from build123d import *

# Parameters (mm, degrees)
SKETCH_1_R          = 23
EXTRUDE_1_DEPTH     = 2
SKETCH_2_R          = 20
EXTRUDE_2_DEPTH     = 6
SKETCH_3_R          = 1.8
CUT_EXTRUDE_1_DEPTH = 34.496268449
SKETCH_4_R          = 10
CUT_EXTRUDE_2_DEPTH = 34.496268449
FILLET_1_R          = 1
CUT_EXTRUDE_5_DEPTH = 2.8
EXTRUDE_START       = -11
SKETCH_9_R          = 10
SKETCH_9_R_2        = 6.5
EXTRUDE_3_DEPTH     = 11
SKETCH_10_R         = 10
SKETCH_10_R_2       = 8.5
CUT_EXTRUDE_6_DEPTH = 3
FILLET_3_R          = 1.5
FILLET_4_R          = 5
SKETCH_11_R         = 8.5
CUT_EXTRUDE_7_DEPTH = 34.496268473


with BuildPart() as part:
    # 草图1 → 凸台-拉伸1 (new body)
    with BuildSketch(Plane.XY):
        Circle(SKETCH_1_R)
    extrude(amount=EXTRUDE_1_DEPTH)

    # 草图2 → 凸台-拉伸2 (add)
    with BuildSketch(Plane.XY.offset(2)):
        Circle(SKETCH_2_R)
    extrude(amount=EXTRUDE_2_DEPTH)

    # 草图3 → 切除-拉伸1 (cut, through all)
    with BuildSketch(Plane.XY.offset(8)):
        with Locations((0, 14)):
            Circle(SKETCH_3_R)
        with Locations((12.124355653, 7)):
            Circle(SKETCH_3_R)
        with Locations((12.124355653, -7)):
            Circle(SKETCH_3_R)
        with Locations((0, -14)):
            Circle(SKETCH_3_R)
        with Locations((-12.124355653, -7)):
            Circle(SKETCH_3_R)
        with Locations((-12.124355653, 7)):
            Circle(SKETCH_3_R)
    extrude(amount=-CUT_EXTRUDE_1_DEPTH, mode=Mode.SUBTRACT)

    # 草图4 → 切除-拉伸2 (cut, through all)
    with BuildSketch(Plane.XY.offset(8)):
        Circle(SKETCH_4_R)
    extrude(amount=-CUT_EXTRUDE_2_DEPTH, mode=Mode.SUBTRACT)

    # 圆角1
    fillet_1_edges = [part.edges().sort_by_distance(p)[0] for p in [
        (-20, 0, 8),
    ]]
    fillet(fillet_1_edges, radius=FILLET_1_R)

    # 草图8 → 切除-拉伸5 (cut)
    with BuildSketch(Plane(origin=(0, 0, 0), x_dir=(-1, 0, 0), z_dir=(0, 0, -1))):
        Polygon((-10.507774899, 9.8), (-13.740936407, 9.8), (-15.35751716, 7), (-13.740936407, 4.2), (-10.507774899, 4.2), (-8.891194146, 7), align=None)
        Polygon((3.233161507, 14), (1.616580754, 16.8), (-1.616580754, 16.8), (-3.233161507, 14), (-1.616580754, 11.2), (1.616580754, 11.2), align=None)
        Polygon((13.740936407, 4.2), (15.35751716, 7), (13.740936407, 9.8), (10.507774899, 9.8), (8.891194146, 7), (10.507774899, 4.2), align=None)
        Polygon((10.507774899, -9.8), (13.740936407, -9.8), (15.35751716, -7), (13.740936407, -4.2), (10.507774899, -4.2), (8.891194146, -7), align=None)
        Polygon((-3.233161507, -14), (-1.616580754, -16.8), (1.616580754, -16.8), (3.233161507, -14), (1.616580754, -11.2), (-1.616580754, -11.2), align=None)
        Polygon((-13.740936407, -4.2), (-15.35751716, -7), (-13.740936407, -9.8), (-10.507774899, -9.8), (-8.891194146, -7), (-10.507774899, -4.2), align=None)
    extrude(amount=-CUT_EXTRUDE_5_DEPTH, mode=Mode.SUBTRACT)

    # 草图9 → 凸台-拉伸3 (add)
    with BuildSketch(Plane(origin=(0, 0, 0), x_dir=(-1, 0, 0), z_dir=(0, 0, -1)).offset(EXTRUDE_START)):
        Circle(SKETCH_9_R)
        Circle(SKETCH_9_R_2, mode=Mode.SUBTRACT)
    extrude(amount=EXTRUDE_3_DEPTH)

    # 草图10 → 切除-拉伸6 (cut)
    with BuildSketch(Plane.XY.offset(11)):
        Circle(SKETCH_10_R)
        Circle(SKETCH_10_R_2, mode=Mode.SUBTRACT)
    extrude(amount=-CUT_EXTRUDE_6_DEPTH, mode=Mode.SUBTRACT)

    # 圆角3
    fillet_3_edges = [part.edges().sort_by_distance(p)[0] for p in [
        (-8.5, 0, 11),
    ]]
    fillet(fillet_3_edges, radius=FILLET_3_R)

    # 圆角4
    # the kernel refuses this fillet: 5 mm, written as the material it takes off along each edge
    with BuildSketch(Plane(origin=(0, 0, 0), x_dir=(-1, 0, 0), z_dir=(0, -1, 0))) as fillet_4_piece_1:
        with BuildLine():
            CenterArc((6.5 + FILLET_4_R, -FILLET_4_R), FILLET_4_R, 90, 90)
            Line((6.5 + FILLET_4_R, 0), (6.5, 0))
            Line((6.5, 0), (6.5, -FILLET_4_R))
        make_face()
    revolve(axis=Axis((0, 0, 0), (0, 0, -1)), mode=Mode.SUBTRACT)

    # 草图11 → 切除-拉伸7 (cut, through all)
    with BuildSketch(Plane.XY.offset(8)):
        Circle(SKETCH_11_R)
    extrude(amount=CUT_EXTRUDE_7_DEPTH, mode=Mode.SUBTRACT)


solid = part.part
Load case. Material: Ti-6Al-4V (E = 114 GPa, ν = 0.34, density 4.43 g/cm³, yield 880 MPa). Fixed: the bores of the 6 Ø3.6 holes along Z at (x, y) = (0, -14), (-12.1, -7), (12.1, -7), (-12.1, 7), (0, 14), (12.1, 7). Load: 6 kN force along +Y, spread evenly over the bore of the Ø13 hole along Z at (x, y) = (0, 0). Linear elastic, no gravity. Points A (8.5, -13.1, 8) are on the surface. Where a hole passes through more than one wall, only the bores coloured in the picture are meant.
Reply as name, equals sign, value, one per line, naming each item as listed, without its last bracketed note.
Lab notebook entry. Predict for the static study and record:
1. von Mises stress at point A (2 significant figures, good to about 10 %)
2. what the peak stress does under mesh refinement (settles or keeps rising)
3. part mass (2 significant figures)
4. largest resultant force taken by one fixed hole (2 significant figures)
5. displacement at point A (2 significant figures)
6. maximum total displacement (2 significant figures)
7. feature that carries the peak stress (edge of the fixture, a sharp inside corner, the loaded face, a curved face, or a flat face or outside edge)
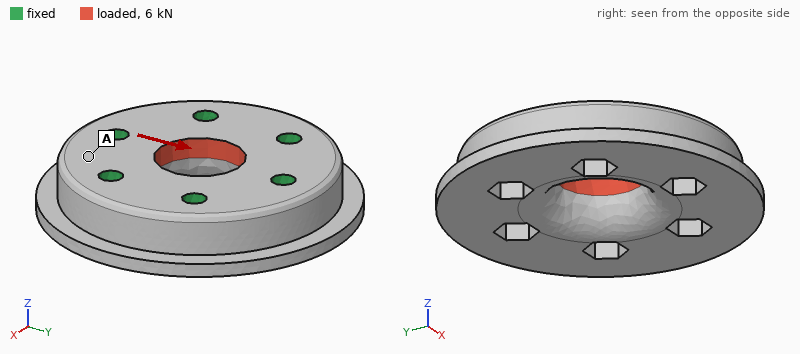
von Mises stress at point A = 8.0 MPa
what the peak stress does under mesh refinement = keeps rising
part mass = 39 g
largest resultant force taken by one fixed hole = 1.5 kN
displacement at point A = 0.75 µm
maximum total displacement = 3.2 µm
feature that carries the peak stress = a sharp inside corner
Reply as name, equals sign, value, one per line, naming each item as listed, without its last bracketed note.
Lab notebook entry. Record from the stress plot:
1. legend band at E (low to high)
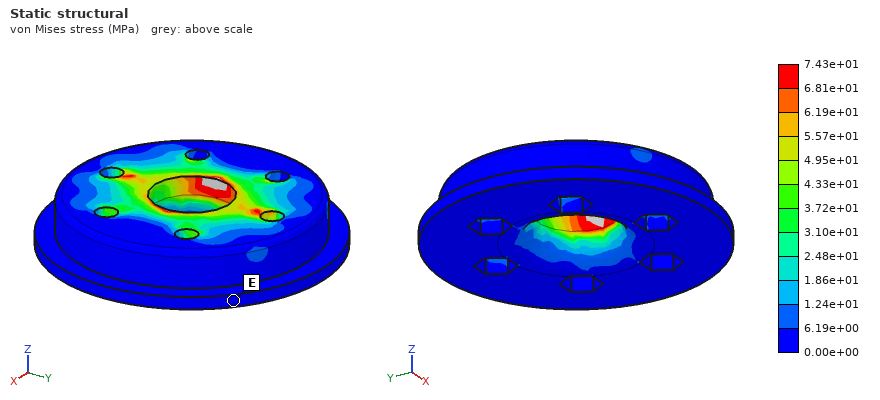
legend band at E = 0.00e+00 to 6.19e+00 MPa
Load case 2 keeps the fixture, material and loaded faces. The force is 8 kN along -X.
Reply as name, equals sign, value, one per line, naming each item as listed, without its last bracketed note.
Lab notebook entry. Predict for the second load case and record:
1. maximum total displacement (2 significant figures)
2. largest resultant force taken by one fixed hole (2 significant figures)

maximum total displacement = 4.6 µm
largest resultant force taken by one fixed hole = 1.7 kN
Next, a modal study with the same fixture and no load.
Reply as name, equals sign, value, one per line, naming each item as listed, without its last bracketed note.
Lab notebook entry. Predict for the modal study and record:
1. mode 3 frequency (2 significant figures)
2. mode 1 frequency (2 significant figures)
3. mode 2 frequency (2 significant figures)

mode 3 frequency = 45 kHz
mode 1 frequency = 45 kHz
mode 2 frequency = 45 kHz
